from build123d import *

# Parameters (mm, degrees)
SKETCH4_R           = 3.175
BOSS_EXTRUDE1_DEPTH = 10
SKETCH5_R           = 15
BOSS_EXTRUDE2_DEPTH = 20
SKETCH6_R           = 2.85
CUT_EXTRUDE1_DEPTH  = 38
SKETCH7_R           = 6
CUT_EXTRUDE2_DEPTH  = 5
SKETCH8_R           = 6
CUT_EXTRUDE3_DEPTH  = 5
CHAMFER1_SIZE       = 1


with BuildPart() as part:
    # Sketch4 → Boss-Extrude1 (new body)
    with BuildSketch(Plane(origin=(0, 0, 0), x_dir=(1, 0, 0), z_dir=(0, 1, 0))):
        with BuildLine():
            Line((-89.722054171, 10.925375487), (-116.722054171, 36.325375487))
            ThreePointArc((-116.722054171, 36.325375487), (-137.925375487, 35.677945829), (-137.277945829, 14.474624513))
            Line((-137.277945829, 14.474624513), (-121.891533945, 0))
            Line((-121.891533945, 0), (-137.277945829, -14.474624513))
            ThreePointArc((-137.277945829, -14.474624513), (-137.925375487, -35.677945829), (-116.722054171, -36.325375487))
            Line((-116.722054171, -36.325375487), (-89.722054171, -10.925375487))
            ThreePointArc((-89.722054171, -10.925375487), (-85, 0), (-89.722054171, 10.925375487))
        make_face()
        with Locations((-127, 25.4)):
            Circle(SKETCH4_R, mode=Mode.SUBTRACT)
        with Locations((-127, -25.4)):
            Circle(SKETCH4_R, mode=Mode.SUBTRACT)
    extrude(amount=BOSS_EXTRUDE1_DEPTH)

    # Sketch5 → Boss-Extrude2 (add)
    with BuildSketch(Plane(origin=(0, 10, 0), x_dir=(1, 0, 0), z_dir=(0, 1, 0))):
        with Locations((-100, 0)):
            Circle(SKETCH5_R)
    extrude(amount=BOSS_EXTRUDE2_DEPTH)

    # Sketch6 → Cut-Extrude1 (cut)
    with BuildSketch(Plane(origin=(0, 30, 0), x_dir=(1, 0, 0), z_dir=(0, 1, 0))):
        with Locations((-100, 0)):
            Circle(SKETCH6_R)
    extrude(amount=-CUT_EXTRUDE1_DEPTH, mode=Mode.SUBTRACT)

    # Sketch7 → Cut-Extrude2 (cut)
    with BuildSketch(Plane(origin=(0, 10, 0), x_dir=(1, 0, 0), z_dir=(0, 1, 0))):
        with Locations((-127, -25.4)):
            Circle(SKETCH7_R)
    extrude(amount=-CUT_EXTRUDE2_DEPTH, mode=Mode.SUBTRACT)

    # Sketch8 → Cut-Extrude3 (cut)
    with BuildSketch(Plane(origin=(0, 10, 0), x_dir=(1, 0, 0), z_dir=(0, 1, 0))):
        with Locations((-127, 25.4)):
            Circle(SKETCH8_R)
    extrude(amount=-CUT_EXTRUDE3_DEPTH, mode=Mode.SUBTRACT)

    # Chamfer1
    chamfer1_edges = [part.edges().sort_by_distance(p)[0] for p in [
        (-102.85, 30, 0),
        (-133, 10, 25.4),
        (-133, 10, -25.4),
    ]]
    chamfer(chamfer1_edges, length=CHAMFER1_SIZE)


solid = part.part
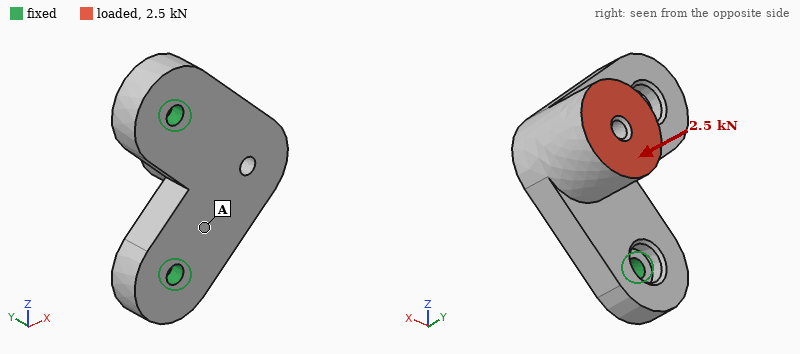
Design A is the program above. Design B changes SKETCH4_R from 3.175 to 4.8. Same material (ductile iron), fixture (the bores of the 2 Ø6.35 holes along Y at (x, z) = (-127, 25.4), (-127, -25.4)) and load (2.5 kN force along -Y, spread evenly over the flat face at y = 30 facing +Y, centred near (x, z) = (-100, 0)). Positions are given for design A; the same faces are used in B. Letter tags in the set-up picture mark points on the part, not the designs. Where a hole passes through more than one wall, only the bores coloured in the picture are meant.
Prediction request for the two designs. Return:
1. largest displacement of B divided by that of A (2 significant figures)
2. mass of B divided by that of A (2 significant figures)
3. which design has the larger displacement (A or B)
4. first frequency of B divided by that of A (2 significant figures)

0.67
0.99
A
1.2
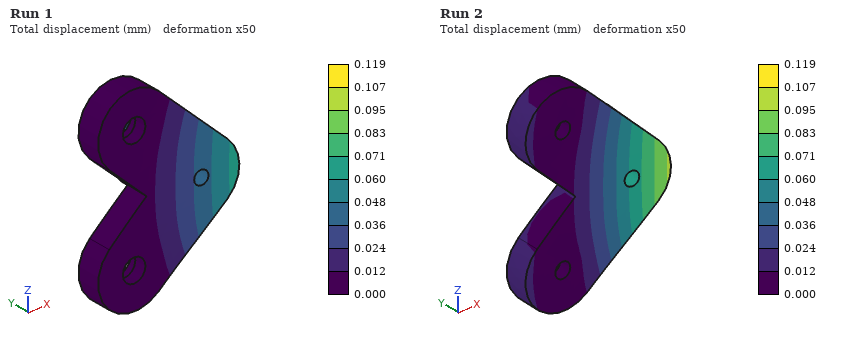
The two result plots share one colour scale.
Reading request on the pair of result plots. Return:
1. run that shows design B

Run 1
